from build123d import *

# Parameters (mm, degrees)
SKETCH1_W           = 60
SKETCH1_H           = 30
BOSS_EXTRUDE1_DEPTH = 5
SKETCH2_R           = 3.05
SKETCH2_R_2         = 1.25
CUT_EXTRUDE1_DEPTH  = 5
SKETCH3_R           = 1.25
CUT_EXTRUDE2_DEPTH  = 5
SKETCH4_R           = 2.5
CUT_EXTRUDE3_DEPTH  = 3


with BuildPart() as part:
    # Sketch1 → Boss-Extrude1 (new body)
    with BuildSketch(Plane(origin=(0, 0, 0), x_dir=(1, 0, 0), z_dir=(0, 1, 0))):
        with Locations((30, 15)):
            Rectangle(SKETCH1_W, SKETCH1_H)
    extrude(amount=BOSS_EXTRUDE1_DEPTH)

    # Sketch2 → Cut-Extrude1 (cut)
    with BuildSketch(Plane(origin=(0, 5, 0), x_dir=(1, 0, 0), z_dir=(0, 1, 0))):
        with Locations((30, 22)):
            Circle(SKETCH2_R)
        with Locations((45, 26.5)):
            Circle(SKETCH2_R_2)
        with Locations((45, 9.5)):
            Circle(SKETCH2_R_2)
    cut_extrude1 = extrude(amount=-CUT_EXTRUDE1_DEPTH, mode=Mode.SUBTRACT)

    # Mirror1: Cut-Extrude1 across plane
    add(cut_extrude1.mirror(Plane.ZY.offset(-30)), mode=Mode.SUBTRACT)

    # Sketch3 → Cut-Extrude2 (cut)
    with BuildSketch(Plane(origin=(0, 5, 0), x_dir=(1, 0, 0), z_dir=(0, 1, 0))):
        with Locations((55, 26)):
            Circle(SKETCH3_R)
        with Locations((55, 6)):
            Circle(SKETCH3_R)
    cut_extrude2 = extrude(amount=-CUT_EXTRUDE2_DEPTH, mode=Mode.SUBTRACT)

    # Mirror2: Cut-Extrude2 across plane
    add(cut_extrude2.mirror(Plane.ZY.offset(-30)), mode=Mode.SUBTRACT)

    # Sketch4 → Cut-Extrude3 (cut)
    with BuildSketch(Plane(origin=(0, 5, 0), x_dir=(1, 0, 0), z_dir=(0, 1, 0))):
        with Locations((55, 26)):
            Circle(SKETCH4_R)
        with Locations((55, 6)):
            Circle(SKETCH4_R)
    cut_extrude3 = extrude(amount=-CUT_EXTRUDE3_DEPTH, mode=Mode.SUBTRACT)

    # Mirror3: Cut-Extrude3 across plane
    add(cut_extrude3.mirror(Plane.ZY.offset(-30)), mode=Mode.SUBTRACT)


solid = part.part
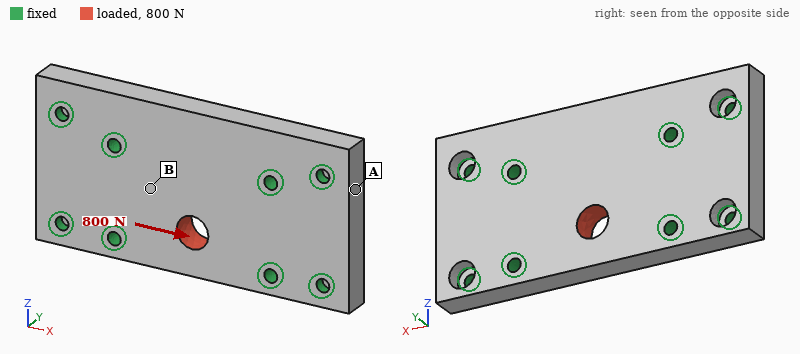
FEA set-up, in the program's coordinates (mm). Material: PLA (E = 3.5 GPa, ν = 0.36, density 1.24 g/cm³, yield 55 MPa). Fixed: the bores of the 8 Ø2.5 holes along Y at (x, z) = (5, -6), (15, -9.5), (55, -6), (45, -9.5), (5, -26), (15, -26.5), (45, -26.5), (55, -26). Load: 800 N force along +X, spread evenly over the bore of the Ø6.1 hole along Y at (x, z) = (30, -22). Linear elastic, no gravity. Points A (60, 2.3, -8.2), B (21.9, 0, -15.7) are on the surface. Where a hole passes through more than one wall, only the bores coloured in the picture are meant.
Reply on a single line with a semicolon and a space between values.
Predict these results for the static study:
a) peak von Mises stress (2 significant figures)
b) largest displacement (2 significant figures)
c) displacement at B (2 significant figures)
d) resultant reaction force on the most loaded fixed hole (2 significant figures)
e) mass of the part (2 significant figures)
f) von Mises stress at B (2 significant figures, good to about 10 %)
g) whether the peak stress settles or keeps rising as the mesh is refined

15 MPa; 27 µm; 9.4 µm; 230 N; 11 g; 3.5 MPa; settles
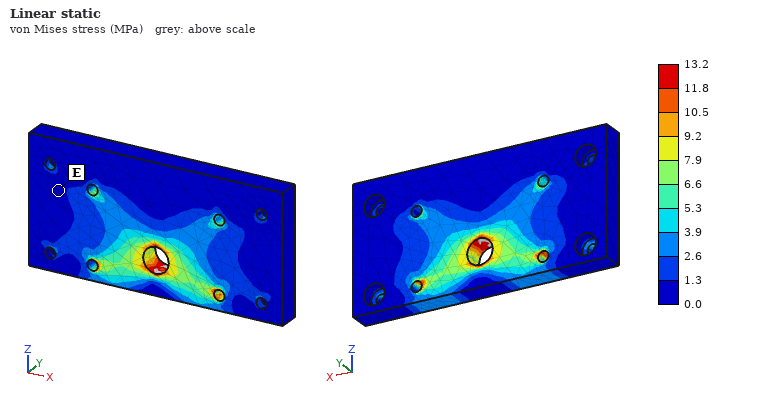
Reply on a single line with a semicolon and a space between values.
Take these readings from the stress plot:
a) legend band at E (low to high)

0.0 to 1.3 MPa
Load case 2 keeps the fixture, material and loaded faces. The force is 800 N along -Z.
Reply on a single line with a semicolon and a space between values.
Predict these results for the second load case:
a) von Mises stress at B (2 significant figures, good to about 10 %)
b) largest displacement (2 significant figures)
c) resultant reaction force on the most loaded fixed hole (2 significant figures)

6.9 MPa; 61 µm; 260 N
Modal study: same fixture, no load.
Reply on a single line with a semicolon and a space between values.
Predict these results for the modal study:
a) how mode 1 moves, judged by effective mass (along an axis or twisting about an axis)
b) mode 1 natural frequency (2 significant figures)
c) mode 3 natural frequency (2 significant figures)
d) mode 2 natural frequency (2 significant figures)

along Y; 7000 Hz; 12 kHz; 8600 Hz
